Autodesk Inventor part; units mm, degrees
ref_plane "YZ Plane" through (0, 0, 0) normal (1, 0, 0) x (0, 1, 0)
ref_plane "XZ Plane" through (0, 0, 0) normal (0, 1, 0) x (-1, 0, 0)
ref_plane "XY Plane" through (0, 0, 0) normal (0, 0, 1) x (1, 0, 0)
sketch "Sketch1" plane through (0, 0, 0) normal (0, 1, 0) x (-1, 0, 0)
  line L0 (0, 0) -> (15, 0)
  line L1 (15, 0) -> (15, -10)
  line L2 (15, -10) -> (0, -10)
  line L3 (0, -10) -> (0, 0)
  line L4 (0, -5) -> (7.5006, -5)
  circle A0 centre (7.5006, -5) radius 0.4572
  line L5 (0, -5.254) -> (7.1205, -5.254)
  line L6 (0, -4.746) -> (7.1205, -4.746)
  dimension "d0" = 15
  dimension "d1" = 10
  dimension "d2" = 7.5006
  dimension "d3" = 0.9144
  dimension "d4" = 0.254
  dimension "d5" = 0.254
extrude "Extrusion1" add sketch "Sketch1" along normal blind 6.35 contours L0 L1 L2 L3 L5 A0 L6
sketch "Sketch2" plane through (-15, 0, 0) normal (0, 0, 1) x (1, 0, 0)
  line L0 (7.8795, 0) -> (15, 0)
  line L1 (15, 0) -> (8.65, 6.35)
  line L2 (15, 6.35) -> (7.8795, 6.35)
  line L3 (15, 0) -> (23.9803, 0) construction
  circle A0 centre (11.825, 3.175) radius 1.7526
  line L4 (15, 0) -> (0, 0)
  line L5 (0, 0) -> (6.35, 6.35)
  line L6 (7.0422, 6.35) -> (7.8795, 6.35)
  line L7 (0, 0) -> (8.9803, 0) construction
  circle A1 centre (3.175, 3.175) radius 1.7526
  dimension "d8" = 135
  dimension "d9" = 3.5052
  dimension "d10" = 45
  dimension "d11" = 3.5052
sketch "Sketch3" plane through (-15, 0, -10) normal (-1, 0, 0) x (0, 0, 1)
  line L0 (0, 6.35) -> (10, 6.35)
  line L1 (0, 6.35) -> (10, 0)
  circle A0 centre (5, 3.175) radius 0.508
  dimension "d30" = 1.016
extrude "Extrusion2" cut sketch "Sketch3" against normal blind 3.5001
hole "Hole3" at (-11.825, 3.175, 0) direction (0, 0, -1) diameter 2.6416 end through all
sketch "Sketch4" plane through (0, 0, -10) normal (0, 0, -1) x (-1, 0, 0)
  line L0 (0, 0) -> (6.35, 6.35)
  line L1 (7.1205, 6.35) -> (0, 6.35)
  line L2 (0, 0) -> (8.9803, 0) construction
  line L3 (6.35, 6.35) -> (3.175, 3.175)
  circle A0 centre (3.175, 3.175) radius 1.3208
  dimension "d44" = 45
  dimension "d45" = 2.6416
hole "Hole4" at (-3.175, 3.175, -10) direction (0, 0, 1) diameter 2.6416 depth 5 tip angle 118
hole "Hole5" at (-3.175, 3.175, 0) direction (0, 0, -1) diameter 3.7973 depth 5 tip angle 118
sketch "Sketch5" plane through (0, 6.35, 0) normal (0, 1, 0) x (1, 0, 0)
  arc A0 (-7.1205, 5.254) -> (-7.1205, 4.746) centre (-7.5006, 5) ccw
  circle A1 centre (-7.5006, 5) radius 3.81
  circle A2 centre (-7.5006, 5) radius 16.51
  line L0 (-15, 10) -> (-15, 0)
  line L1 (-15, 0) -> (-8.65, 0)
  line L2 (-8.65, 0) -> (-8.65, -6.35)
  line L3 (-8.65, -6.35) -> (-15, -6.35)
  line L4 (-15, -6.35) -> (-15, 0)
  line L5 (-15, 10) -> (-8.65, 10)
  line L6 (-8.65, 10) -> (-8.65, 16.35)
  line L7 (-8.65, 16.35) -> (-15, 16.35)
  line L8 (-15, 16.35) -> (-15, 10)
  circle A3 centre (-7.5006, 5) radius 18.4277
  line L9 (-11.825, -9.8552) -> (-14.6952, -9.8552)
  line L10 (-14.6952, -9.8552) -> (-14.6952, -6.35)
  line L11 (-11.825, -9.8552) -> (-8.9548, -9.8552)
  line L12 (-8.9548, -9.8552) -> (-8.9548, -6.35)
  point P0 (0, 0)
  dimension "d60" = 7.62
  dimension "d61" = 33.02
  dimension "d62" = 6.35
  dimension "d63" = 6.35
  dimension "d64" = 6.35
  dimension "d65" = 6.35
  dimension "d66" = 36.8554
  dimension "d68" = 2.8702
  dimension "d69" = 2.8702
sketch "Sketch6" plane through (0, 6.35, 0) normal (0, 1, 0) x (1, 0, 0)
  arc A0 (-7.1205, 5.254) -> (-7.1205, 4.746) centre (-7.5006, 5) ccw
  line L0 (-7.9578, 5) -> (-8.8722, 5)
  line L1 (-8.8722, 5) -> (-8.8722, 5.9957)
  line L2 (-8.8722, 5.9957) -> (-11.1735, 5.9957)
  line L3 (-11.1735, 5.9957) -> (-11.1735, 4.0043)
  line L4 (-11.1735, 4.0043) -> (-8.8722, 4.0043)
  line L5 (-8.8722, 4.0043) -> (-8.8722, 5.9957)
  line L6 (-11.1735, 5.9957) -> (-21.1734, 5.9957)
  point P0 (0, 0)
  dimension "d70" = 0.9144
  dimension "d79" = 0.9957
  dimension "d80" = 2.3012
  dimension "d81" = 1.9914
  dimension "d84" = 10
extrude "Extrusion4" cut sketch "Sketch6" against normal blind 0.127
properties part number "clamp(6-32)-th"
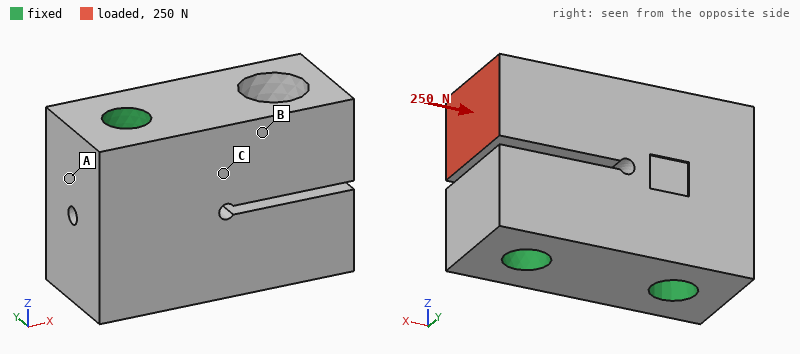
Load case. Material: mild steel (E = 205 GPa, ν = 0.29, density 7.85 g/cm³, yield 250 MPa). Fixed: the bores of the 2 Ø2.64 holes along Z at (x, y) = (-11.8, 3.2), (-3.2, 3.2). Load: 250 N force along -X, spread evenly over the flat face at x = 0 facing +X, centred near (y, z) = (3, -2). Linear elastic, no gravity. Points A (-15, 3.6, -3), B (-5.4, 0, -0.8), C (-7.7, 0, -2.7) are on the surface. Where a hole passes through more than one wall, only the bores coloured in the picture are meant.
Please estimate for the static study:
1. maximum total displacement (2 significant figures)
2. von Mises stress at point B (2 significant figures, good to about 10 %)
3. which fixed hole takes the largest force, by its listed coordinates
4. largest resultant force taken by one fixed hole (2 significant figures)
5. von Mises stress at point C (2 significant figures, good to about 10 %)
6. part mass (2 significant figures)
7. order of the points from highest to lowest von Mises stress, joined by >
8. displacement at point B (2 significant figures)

1.3 µm
22 MPa
(-11.8, 3.2)
240 N
13 MPa
6.2 g
B > C > A
0.46 µm
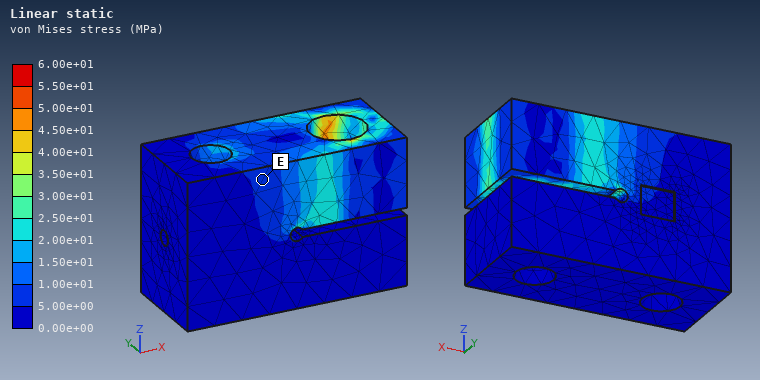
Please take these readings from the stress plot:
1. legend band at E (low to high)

5.00e+00 to 1.00e+01 MPa
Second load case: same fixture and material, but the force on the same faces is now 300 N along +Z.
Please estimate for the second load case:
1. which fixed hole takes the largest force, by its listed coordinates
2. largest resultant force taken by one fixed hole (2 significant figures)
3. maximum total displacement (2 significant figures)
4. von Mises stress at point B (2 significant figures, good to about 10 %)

(-11.8, 3.2)
290 N
14 µm
77 MPa
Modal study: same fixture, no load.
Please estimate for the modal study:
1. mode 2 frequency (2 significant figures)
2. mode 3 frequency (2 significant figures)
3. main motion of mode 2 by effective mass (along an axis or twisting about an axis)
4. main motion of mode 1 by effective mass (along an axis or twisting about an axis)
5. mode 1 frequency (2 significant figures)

36 kHz
65 kHz
along Z
along Y
33 kHz
